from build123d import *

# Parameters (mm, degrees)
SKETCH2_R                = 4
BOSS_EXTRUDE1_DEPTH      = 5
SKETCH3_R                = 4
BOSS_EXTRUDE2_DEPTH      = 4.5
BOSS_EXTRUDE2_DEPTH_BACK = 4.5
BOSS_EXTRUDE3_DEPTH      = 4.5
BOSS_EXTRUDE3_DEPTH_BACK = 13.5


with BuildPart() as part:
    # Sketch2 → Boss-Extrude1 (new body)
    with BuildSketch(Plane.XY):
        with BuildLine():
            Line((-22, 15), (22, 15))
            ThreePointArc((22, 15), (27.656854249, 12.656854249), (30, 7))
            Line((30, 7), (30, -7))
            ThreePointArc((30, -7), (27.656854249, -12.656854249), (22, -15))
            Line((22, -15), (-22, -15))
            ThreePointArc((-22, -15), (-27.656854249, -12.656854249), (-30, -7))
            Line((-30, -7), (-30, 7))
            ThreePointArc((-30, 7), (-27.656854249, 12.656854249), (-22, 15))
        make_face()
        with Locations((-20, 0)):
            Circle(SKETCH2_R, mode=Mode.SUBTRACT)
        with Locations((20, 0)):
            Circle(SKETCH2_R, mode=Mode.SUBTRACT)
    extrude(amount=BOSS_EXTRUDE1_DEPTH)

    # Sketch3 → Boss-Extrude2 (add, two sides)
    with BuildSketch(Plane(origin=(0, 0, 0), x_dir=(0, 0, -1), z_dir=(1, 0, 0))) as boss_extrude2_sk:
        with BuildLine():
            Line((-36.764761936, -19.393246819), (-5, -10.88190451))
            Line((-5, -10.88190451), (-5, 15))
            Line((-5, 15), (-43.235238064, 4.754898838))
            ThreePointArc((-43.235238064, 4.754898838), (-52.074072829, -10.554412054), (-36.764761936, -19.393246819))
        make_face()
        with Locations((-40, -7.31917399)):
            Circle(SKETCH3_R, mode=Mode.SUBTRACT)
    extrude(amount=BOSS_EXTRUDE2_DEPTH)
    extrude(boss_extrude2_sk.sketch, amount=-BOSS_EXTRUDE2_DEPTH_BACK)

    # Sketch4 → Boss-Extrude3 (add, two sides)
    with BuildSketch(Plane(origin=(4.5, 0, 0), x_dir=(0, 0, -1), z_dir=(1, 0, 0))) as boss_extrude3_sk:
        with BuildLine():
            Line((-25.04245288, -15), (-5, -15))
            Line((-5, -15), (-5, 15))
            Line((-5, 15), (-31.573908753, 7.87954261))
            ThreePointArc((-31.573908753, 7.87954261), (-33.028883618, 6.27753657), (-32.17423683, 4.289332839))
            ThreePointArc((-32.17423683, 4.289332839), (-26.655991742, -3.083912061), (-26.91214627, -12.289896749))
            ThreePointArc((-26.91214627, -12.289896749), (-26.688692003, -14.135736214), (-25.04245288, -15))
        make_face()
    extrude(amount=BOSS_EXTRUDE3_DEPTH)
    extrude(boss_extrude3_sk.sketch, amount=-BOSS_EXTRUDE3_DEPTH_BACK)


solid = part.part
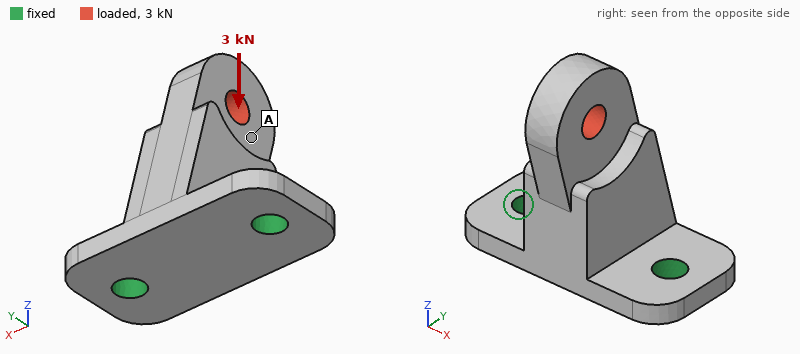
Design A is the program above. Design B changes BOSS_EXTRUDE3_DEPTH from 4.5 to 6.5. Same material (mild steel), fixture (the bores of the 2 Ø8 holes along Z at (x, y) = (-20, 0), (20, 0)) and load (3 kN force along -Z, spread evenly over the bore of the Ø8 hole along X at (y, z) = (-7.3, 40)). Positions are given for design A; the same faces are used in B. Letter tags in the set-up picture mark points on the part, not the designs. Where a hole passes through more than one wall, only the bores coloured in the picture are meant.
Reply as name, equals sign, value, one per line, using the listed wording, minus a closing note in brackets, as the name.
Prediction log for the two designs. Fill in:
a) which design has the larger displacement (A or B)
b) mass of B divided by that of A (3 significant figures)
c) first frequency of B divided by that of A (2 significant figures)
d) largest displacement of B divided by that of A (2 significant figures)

which design has the larger displacement = A
mass of B divided by that of A = 1.05
first frequency of B divided by that of A = 1.0
largest displacement of B divided by that of A = 0.91
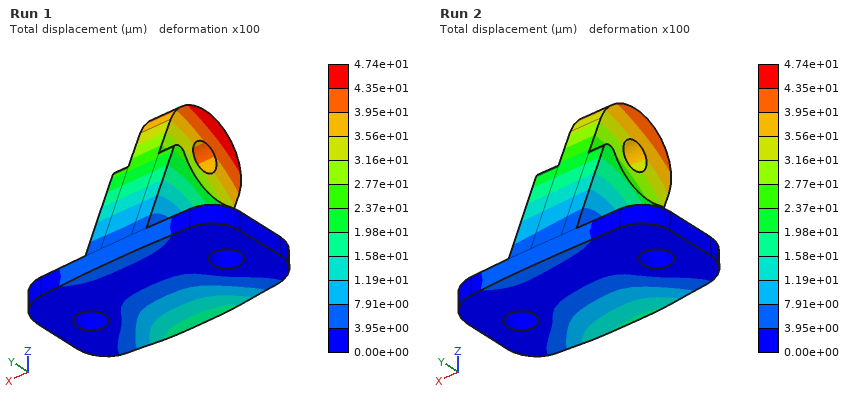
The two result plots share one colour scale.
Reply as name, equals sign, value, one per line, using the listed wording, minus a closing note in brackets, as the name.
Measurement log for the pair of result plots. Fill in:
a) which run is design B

which run is design B = Run 2
